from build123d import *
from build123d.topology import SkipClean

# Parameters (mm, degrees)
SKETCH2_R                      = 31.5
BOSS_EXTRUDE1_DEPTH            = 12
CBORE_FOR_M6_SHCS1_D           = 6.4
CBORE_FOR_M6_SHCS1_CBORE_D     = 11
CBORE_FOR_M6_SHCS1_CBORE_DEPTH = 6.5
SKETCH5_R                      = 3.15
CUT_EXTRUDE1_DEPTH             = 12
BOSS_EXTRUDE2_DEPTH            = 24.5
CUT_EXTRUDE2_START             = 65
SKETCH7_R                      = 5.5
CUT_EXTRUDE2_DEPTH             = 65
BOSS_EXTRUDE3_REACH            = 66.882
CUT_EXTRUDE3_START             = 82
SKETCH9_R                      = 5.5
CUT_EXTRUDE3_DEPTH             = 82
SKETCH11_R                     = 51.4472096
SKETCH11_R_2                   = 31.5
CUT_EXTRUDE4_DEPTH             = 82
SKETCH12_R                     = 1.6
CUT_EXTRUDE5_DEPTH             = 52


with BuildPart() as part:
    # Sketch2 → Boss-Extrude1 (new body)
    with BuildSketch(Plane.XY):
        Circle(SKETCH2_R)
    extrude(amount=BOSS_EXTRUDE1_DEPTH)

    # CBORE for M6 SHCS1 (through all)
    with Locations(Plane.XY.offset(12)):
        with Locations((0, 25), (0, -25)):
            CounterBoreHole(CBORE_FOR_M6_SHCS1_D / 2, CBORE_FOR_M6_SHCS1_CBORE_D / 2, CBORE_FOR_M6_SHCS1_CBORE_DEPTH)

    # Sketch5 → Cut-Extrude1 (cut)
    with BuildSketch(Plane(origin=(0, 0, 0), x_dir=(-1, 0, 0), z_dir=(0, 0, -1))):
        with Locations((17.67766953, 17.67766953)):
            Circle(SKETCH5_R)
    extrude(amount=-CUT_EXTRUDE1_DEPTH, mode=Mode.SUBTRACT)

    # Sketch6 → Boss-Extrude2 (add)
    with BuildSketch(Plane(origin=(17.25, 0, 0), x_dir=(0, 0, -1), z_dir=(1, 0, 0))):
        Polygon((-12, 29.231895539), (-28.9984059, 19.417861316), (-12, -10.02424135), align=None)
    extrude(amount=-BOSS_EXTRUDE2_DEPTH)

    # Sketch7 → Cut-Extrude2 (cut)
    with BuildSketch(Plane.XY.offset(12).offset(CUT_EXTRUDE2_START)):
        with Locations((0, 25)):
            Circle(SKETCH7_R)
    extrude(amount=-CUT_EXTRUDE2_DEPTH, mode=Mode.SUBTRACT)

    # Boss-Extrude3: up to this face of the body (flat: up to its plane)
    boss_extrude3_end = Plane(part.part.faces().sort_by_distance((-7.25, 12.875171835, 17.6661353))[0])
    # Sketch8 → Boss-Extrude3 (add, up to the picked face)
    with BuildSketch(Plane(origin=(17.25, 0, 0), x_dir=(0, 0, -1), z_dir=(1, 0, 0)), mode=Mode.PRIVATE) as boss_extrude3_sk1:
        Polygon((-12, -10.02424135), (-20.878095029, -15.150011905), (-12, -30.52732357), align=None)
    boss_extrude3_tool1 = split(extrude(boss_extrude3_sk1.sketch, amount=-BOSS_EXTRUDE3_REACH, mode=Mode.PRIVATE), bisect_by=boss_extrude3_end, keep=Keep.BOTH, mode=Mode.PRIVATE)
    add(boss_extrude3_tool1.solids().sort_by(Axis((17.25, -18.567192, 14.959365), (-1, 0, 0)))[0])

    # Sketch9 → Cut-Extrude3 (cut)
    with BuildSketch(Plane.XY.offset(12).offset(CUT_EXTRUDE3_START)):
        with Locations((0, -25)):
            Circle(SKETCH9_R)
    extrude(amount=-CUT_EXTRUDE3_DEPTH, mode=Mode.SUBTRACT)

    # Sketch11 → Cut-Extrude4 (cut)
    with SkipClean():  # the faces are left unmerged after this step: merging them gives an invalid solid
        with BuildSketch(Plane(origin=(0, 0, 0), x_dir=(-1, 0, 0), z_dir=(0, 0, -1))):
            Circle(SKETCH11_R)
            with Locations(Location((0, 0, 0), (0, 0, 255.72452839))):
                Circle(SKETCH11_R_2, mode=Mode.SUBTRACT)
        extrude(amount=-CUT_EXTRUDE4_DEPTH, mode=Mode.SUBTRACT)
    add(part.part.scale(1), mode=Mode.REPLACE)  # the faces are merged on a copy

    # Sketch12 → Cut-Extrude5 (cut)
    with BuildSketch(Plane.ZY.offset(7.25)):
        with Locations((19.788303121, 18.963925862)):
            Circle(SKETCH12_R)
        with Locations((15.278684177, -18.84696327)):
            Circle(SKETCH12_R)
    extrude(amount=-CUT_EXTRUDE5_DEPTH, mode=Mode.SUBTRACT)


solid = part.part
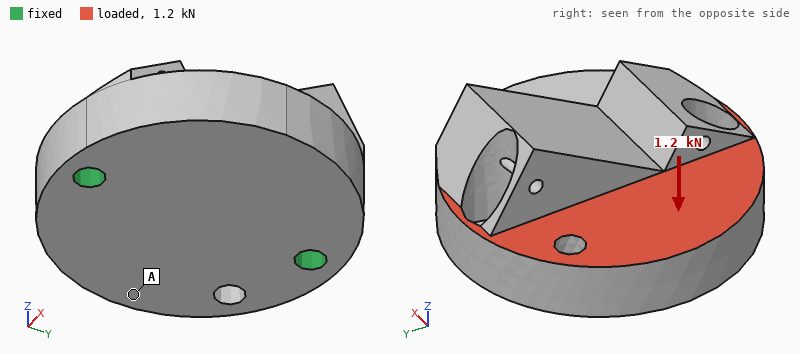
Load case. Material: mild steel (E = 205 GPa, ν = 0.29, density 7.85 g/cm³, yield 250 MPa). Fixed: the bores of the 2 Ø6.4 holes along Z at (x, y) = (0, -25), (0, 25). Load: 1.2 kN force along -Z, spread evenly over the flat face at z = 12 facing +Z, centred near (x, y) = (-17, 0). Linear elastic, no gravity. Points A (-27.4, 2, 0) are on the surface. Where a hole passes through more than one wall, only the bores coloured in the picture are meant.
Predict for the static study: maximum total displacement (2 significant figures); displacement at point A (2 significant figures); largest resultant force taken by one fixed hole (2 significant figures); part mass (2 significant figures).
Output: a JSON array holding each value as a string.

["13 µm", "11 µm", "690 N", "350 g"]
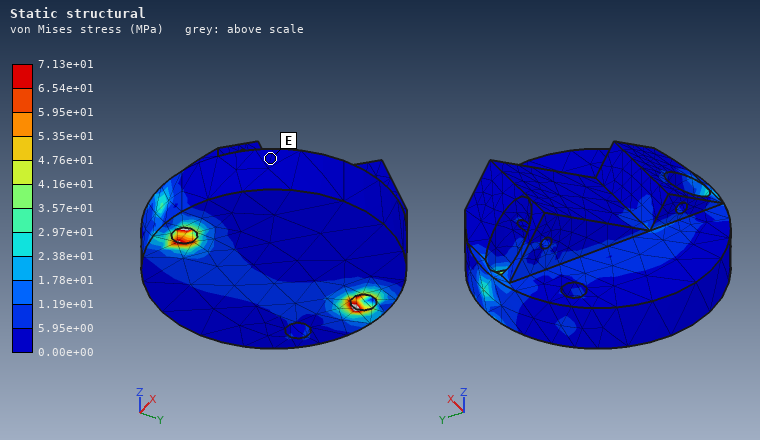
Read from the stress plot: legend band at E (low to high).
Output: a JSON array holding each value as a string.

["0.00e+00 to 5.95e+00 MPa"]
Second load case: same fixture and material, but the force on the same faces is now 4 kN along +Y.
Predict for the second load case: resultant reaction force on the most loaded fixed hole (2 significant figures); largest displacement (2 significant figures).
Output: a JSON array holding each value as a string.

["2.5 kN", "3.1 µm"]
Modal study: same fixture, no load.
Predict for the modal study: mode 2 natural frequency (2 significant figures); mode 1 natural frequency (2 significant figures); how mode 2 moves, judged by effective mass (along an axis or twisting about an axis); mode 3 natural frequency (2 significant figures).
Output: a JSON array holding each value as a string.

["9400 Hz", "4100 Hz", "along Z", "16 kHz"]
